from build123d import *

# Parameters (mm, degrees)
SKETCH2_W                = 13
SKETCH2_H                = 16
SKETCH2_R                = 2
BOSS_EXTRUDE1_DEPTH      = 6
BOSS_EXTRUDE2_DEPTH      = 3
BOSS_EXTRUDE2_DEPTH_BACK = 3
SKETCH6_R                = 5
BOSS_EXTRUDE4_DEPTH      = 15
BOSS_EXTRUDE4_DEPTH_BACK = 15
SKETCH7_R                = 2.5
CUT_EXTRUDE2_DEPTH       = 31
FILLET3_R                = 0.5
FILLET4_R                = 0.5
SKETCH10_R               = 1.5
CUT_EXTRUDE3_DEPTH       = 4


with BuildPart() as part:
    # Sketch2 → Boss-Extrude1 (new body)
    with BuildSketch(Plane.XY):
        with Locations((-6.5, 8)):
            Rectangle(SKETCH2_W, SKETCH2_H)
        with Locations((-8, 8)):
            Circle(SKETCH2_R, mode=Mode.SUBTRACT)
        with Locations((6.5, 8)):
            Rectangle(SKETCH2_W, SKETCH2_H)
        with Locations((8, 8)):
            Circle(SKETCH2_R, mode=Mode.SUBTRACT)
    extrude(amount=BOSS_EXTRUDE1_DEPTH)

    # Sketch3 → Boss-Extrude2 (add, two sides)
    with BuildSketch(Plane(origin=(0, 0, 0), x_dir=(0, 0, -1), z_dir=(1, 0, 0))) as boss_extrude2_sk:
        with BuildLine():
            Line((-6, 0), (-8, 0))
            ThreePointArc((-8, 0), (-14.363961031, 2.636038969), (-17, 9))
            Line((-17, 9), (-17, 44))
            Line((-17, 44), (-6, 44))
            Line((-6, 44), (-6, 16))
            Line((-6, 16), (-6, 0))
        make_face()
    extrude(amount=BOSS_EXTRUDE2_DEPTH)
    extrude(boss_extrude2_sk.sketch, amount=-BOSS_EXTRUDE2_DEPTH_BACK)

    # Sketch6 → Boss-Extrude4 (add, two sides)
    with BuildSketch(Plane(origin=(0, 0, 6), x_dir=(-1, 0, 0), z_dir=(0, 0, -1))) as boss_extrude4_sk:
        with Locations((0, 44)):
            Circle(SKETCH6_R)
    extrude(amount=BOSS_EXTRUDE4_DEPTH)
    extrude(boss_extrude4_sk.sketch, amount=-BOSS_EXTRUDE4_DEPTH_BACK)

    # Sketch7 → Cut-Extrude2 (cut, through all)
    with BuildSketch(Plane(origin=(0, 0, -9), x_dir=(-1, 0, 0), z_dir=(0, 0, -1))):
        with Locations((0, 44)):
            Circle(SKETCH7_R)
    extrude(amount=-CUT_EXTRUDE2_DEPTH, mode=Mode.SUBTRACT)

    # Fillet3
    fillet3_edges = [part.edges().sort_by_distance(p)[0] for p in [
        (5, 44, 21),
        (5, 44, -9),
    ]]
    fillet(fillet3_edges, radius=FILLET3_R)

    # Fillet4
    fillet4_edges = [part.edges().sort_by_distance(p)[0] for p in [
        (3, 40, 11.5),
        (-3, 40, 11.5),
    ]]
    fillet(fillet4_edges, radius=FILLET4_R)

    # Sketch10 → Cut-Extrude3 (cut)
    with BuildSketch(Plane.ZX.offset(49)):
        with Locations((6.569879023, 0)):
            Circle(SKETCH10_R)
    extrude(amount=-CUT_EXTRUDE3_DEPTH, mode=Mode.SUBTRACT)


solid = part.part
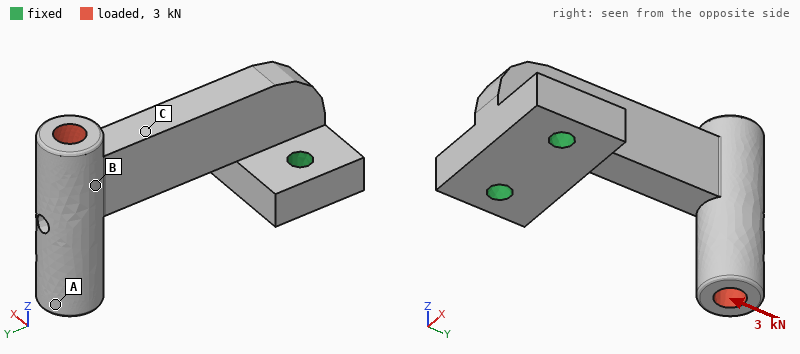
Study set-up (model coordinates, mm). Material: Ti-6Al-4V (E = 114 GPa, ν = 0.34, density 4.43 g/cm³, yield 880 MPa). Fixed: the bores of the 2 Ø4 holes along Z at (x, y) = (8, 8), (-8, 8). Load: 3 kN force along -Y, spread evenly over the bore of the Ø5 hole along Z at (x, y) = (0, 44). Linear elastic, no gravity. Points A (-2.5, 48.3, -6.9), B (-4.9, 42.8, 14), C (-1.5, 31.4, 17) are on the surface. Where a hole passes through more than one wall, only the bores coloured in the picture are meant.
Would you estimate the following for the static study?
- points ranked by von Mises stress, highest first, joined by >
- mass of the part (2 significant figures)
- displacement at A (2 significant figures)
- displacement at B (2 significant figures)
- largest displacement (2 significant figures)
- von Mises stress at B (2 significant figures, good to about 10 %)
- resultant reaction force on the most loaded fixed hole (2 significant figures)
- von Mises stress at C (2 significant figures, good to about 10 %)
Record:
C > B > A
29 g
0.20 mm
0.073 mm
0.21 mm
44 MPa
1.5 kN
94 MPa
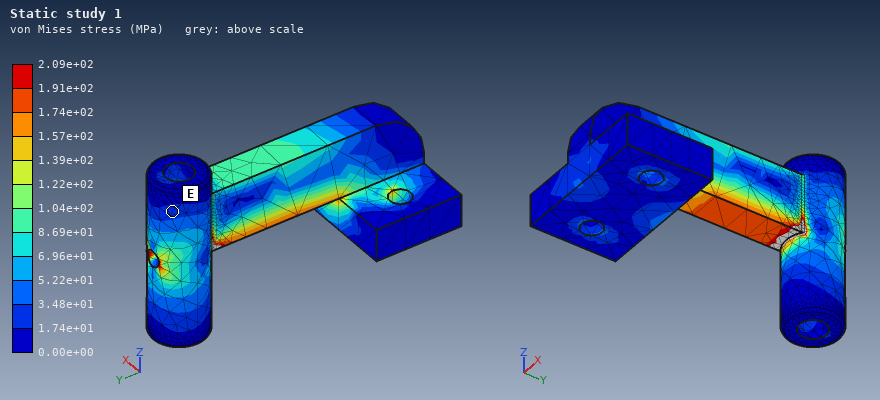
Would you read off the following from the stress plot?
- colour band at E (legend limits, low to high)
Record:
1.74e+01 to 3.48e+01 MPa
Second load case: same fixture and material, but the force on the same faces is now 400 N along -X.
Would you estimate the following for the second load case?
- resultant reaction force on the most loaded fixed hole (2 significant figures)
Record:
840 N
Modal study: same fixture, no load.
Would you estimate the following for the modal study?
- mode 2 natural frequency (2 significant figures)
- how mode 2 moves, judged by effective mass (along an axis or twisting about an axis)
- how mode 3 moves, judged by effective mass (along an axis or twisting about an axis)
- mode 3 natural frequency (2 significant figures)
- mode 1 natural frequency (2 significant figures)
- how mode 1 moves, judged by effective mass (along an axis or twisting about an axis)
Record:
3000 Hz
along Z
twisting about Y
4900 Hz
2200 Hz
along X
